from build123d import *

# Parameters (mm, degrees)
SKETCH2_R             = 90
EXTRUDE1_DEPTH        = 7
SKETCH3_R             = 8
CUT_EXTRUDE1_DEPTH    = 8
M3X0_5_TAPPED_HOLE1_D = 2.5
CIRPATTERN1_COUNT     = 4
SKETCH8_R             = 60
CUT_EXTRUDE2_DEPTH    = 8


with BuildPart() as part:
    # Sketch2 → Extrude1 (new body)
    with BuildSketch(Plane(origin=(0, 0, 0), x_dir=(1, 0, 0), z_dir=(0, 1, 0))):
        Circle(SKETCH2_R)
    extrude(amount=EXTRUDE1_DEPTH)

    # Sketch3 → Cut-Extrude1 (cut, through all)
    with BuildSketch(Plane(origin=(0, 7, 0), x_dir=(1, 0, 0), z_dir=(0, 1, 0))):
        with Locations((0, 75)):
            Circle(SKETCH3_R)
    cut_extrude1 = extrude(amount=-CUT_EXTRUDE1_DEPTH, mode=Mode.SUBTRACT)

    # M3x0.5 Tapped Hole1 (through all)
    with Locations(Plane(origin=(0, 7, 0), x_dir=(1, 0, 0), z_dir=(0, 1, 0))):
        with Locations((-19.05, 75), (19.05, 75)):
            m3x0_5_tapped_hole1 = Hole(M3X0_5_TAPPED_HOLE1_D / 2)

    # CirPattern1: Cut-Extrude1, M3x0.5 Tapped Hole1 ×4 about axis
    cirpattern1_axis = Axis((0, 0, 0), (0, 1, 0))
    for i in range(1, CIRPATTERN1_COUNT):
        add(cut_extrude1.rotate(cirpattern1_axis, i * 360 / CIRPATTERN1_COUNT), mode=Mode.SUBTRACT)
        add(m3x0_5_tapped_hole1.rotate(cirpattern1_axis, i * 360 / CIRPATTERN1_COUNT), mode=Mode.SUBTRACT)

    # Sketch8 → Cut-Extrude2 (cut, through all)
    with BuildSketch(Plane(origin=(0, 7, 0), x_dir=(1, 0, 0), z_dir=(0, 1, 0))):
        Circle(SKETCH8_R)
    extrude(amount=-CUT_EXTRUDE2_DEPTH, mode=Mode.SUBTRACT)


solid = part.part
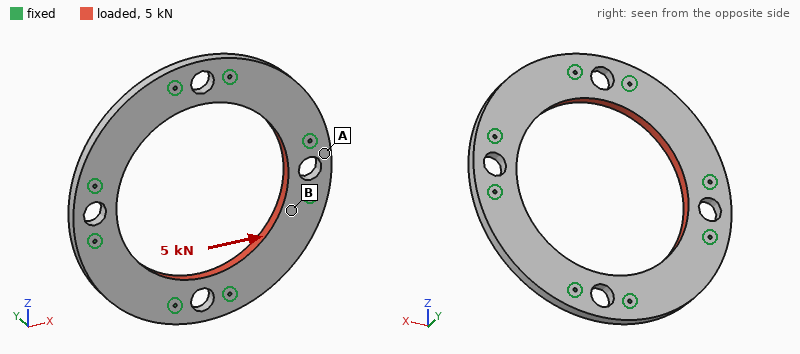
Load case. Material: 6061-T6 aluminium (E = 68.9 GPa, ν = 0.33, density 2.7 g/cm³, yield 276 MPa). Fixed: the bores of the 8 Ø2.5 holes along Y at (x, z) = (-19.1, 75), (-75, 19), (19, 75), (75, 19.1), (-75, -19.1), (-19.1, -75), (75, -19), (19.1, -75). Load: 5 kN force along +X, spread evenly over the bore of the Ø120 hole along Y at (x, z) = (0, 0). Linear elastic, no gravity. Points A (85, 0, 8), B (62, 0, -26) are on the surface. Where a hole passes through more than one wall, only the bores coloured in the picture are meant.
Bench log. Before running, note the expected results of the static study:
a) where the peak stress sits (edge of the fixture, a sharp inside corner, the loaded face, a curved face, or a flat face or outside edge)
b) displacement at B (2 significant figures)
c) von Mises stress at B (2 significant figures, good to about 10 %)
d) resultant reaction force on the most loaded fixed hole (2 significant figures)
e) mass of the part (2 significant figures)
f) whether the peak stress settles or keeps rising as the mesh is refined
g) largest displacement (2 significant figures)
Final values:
edge of the fixture
1.9 µm
4.2 MPa
660 N
250 g
keeps rising
3.9 µm
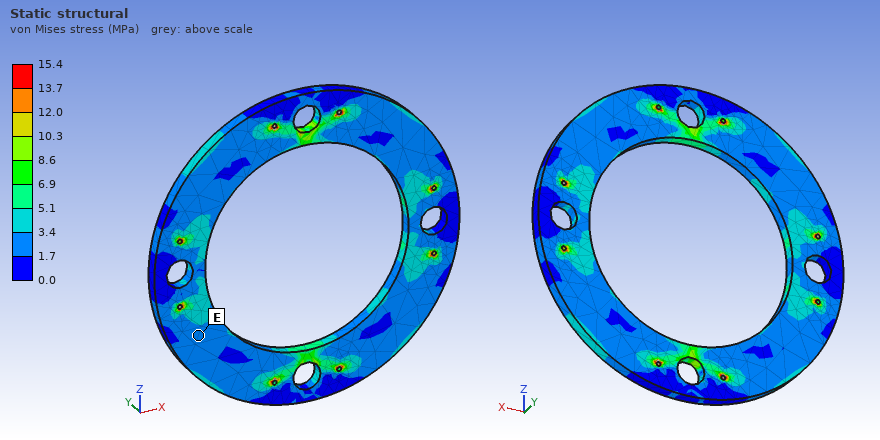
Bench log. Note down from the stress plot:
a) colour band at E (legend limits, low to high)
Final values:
1.7 to 3.4 MPa
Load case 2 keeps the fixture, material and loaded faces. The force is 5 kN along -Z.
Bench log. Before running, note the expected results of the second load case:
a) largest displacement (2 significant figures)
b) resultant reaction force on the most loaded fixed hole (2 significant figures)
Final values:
3.9 µm
660 N
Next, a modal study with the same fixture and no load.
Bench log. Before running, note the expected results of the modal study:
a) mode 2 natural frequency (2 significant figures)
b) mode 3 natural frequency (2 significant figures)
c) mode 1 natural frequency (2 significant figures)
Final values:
4200 Hz
4200 Hz
4100 Hz
